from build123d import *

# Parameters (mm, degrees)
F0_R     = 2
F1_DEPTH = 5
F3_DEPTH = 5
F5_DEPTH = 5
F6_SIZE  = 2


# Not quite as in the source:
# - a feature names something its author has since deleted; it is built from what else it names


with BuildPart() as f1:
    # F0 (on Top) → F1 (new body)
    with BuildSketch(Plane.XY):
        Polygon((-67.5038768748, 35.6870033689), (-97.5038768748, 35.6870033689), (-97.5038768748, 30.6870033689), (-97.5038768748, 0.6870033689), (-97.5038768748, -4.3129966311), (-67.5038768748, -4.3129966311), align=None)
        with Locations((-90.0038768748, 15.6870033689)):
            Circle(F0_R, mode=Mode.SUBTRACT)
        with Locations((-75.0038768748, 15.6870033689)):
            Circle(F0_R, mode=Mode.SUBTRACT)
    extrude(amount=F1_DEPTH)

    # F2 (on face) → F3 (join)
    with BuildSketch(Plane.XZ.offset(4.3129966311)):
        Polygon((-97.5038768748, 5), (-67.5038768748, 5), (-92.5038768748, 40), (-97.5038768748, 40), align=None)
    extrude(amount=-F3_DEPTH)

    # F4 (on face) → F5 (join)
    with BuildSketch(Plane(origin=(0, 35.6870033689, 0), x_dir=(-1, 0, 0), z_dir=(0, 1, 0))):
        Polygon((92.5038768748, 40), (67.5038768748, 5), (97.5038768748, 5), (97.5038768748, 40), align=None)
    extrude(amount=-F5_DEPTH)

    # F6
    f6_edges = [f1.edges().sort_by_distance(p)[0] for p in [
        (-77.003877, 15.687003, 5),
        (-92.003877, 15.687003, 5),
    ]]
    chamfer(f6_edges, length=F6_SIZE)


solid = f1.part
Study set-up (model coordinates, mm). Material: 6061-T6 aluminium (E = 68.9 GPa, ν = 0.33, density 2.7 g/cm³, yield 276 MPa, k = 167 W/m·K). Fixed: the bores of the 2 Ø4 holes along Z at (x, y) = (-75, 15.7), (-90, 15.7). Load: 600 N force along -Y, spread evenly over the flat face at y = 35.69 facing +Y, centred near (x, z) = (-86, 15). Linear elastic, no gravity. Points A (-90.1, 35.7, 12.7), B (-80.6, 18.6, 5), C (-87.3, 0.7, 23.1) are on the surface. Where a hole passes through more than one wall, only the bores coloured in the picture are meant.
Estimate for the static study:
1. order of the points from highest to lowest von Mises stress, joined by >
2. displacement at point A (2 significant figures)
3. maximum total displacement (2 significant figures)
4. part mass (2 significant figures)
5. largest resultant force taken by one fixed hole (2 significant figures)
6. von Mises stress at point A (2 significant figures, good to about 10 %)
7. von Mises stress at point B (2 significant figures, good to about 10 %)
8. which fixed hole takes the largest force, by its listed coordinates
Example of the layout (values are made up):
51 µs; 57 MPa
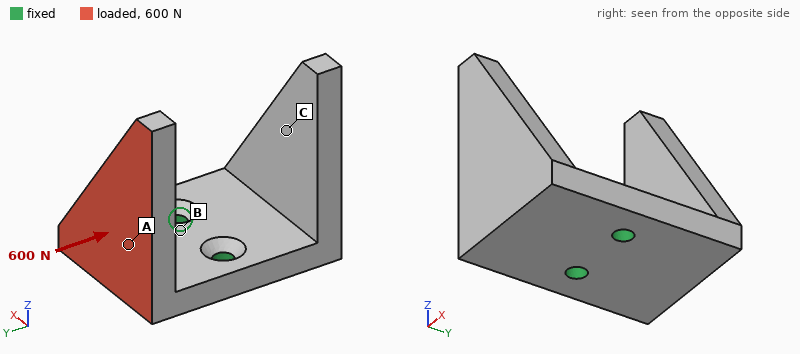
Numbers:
B > A > C; 0.13 mm; 0.42 mm; 32 g; 430 N; 33 MPa; 59 MPa; (-90, 15.7)
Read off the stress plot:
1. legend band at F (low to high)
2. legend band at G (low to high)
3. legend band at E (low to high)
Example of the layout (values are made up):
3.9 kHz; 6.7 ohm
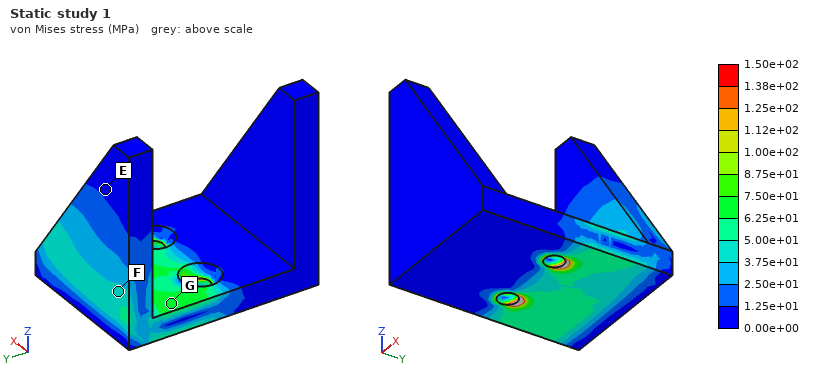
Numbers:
3.75e+01 to 5.00e+01 MPa; 6.25e+01 to 7.50e+01 MPa; 0.00e+00 to 1.25e+01 MPa
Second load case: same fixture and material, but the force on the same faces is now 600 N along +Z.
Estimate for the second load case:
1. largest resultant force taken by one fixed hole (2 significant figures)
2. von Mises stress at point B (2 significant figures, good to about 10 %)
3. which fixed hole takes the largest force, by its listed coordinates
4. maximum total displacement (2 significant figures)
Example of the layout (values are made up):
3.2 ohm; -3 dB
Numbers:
430 N; 72 MPa; (-90, 15.7); 0.32 mm
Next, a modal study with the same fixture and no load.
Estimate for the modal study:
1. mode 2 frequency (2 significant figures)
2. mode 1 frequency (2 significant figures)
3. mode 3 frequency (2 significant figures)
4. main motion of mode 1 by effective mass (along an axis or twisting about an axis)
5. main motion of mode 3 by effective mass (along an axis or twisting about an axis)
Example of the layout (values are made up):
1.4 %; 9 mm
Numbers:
2500 Hz; 2200 Hz; 4300 Hz; along Y; twisting about Z
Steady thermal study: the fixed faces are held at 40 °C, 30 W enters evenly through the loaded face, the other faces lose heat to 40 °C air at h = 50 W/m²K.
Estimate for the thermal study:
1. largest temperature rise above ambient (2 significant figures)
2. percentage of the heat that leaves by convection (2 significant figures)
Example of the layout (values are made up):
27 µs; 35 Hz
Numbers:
40 K; 8.4 %
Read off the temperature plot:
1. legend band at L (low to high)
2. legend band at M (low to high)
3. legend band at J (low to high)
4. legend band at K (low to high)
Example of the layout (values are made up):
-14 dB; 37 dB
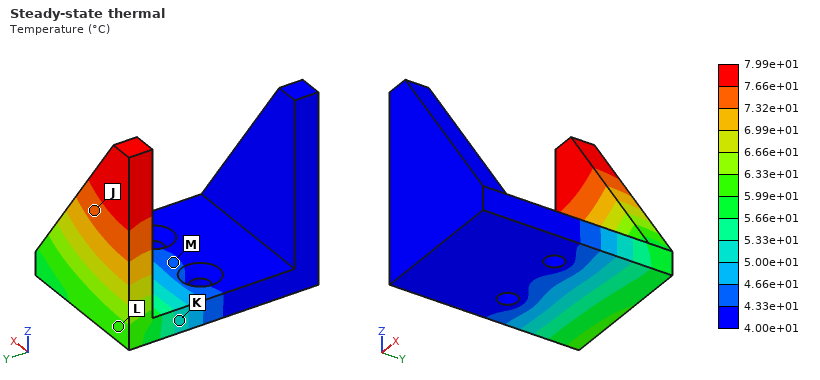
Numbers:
5.99e+01 to 6.33e+01 °C; 4.33e+01 to 4.66e+01 °C; 7.32e+01 to 7.66e+01 °C; 5.00e+01 to 5.33e+01 °C
